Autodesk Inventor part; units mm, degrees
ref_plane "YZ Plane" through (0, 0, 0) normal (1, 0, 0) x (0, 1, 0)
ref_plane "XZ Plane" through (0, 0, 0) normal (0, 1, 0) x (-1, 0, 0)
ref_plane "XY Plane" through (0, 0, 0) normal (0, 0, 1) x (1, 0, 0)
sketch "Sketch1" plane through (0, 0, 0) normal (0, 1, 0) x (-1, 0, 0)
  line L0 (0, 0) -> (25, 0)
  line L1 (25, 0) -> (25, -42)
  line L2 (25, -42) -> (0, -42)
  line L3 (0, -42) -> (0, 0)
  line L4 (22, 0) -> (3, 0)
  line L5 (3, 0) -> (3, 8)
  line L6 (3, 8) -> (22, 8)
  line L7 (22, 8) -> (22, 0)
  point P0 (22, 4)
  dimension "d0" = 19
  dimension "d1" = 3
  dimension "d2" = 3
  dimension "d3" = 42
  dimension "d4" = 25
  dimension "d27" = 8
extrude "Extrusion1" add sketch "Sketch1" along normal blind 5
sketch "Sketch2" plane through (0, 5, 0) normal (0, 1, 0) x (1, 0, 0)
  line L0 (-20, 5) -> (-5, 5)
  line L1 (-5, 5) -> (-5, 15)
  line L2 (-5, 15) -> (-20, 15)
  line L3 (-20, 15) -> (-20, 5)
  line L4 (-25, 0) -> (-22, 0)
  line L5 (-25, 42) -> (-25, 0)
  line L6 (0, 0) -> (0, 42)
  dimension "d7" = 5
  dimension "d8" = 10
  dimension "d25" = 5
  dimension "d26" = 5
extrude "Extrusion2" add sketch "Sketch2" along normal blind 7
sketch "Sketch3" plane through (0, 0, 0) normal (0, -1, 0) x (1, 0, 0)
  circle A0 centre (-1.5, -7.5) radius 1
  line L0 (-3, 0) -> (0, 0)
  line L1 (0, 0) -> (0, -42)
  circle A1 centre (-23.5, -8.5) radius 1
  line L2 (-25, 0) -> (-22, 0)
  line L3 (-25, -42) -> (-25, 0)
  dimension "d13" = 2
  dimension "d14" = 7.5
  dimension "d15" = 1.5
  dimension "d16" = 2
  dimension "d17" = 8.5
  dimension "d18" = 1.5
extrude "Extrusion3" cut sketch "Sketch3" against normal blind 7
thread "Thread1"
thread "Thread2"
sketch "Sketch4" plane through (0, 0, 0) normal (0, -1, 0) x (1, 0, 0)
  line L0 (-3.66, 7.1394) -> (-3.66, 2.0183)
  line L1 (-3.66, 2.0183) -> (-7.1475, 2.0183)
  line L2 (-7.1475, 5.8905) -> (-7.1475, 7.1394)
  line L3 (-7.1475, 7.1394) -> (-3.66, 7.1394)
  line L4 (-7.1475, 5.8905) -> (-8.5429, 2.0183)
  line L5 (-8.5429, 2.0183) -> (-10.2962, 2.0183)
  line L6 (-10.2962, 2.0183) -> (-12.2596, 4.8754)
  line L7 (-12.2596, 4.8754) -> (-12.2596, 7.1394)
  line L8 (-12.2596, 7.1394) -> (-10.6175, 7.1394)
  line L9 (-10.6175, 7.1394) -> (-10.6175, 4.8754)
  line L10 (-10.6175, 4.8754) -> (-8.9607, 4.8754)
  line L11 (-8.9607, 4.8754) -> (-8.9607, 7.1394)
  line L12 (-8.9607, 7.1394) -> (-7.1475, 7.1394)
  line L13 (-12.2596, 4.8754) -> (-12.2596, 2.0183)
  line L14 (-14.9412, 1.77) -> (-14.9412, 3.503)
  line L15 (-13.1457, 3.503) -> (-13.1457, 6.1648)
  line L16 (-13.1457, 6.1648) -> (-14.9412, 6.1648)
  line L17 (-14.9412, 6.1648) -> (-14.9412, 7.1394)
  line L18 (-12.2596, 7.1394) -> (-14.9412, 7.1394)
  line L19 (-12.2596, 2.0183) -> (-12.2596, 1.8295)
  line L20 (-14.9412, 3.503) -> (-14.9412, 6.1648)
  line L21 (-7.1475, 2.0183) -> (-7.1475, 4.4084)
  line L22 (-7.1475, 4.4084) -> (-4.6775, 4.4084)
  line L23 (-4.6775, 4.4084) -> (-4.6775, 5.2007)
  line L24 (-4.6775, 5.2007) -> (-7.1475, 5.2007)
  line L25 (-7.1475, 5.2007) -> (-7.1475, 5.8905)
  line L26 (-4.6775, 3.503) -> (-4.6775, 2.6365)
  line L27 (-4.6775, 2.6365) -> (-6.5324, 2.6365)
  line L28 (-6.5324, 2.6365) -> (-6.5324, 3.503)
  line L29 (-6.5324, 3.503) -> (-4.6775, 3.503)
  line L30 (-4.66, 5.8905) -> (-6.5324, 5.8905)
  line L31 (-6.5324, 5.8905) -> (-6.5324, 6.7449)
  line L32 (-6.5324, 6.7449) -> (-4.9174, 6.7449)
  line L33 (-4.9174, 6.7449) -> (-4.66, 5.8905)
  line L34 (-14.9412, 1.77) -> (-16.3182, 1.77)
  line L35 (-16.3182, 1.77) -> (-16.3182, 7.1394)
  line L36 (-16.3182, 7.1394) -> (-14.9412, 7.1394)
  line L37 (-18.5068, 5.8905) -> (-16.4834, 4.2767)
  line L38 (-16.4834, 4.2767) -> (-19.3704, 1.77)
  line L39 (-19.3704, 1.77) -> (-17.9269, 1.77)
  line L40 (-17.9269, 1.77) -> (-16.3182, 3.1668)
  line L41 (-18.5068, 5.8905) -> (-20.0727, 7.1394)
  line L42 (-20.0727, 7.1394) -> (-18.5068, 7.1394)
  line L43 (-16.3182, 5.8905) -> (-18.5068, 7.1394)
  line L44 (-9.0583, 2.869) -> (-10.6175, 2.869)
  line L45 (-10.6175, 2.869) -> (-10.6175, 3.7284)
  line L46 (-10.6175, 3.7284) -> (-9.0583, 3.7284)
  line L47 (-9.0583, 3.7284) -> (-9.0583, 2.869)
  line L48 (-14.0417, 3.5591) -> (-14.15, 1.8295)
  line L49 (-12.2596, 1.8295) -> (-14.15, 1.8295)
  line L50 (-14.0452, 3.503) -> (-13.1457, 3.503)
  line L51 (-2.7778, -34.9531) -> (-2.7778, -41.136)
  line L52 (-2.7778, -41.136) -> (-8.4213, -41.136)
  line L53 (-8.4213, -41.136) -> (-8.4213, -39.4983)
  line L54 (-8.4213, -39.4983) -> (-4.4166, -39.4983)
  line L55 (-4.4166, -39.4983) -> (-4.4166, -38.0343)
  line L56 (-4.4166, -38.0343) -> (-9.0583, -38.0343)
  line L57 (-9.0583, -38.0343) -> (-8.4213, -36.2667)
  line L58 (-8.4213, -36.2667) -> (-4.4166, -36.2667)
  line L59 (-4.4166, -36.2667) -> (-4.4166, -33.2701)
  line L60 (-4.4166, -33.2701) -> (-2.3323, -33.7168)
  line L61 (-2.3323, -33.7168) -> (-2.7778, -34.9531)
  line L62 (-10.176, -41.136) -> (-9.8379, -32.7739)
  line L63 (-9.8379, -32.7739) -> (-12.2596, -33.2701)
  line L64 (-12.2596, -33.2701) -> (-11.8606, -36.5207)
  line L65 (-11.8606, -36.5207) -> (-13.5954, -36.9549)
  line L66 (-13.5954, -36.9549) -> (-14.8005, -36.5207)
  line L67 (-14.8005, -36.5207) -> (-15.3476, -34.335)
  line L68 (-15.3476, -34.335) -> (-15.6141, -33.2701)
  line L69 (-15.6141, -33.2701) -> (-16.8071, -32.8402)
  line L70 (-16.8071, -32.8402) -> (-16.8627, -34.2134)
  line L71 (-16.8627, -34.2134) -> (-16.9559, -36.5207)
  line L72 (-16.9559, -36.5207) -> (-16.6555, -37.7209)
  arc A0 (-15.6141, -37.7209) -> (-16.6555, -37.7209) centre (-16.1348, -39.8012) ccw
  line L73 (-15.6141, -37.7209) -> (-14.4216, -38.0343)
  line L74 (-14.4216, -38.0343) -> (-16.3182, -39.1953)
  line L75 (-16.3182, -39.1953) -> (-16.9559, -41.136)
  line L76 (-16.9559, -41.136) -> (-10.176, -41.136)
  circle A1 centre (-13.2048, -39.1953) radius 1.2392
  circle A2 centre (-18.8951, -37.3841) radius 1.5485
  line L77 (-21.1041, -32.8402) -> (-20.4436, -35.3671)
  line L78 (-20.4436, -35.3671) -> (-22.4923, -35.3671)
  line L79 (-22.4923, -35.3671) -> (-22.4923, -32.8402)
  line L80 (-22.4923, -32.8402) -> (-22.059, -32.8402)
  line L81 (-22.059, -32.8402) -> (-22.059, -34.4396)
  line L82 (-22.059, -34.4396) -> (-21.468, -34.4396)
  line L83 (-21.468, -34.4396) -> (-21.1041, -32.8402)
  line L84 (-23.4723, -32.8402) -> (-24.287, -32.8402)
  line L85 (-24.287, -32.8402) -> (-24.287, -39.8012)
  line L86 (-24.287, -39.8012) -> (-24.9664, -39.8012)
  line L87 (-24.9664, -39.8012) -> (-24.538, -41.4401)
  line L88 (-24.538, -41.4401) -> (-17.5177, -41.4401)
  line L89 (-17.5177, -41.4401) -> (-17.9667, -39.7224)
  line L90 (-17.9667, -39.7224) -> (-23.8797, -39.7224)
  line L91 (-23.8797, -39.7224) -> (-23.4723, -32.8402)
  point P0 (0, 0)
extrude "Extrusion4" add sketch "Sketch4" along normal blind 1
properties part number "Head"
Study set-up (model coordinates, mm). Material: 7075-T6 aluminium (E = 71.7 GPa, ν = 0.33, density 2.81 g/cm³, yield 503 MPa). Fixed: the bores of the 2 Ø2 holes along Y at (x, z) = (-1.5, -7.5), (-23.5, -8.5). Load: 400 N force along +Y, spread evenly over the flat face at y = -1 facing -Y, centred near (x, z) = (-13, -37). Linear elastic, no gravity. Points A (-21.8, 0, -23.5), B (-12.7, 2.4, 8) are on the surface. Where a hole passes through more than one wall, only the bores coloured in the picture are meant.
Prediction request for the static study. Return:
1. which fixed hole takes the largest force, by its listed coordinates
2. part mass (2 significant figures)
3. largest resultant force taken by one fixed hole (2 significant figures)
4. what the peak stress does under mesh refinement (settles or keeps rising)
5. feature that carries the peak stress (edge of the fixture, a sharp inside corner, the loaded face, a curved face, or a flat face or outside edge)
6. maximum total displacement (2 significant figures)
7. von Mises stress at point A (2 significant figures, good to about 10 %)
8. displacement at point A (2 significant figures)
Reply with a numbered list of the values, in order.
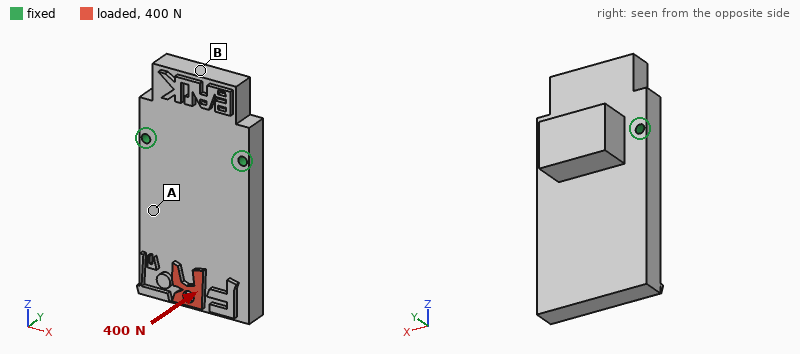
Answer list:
1. (-23.5, -8.5)
2. 20 g
3. 270 N
4. keeps rising
5. edge of the fixture
6. 0.25 mm
7. 55 MPa
8. 0.077 mm
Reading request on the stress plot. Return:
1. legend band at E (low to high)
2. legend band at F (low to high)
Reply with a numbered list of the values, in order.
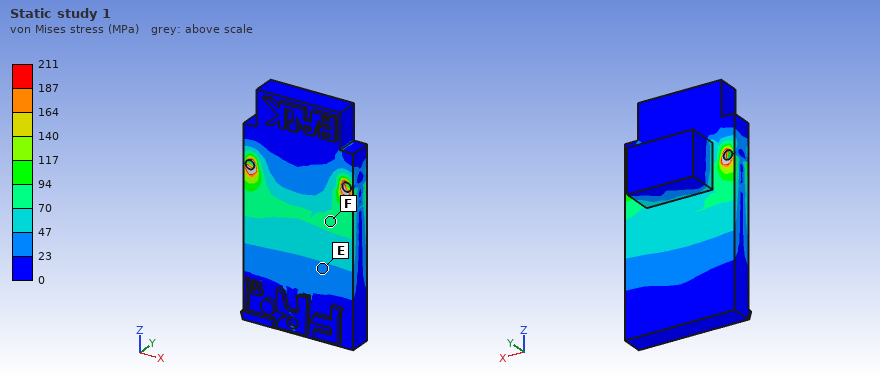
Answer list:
1. 23 to 47 MPa
2. 70 to 94 MPa
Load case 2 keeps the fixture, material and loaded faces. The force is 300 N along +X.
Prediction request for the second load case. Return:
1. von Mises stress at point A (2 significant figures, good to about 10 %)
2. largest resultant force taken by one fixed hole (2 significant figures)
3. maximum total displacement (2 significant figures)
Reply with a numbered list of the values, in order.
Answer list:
1. 11 MPa
2. 430 N
3. 17 µm
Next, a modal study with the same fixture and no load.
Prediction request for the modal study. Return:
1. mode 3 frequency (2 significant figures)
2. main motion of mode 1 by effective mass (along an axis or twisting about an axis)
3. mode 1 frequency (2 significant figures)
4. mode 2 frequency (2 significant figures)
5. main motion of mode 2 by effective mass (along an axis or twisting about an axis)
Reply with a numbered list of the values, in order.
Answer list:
1. 13 kHz
2. along Y
3. 3100 Hz
4. 10 kHz
5. twisting about Z
